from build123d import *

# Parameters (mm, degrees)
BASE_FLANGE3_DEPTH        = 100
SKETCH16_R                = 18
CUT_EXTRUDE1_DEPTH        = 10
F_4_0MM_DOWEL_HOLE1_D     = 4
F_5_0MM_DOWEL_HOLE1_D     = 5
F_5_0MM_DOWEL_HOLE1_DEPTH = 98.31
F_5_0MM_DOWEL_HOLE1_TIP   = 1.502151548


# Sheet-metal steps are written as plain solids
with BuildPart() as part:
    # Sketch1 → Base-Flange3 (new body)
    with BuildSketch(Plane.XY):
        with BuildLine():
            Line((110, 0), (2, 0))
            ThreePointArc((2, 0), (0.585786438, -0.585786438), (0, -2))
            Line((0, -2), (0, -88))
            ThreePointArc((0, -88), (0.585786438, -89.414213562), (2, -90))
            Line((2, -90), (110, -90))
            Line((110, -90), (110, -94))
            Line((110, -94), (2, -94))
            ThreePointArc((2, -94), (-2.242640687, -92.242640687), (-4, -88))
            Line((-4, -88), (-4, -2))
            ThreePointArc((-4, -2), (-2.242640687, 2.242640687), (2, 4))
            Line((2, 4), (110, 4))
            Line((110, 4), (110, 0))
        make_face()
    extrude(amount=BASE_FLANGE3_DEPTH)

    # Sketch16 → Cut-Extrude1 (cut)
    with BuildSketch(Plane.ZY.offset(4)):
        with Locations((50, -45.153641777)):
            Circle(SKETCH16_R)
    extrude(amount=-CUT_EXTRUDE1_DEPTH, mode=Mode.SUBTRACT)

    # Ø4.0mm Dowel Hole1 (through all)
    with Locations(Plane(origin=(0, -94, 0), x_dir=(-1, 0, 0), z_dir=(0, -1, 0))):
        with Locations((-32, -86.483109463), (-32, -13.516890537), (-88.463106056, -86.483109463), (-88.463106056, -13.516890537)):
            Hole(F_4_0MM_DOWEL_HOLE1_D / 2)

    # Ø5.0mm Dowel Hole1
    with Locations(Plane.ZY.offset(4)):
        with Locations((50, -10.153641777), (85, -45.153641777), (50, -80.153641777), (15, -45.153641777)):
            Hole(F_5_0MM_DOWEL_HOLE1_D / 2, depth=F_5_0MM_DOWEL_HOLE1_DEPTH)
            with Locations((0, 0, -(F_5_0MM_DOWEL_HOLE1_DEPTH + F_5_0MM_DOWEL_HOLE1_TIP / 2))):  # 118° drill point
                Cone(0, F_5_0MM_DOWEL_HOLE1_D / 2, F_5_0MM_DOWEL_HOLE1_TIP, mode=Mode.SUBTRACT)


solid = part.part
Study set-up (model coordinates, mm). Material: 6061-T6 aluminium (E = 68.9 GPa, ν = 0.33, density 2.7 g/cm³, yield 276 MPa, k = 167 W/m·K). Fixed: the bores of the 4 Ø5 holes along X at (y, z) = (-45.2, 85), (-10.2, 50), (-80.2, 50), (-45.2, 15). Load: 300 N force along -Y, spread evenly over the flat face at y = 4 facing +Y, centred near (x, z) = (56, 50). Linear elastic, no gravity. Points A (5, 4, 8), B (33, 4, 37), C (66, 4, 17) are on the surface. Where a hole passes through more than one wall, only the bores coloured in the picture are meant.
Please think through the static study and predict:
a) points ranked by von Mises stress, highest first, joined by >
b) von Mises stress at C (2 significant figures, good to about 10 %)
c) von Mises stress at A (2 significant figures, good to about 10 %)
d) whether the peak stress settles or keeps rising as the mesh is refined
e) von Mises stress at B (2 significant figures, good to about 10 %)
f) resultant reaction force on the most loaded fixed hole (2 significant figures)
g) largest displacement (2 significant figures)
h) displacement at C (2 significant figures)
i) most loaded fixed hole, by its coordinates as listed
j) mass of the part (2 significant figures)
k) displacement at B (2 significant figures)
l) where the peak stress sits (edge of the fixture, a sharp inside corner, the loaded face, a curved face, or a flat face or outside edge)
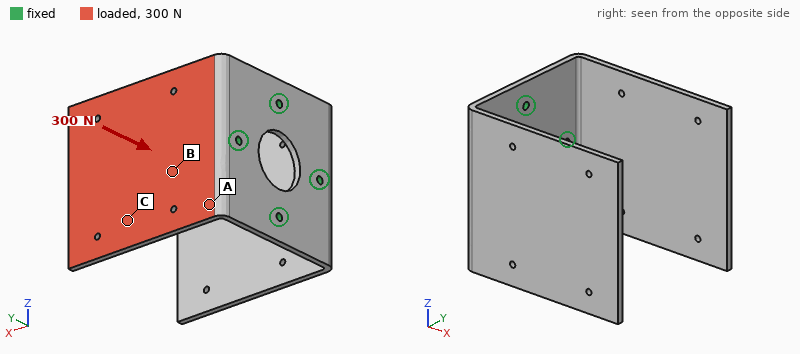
A > B > C
10 MPa
46 MPa
keeps rising
29 MPa
350 N
2.1 mm
1.1 mm
(-10.2, 50)
330 g
0.45 mm
edge of the fixture
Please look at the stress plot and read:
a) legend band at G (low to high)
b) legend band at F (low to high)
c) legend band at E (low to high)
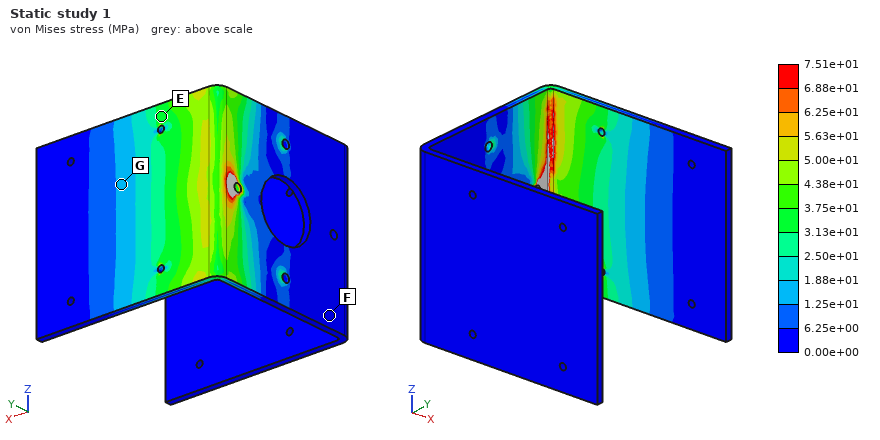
1.25e+01 to 1.88e+01 MPa
0.00e+00 to 6.25e+00 MPa
3.13e+01 to 3.75e+01 MPa
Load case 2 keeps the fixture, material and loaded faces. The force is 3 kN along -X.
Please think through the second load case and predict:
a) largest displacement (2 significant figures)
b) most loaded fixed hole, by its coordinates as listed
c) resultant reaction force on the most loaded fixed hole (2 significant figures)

2.1 mm
(-10.2, 50)
3.4 kN
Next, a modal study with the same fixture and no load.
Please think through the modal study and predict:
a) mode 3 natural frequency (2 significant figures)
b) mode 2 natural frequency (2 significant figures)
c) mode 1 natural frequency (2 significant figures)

400 Hz
220 Hz
220 Hz
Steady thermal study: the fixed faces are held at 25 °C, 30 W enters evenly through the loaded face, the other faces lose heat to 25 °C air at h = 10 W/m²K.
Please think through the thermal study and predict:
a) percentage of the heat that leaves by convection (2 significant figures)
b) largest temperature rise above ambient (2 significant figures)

13 %
34 K
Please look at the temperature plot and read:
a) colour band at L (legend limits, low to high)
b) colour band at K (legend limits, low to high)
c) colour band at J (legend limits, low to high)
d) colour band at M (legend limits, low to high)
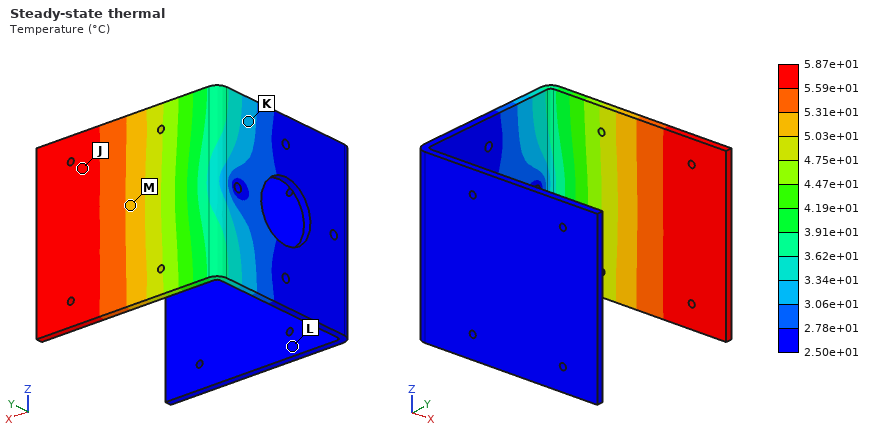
2.50e+01 to 2.78e+01 °C
3.06e+01 to 3.34e+01 °C
5.59e+01 to 5.87e+01 °C
5.03e+01 to 5.31e+01 °C
